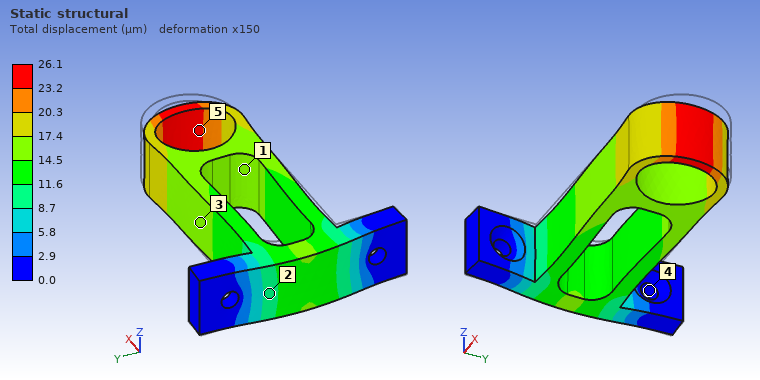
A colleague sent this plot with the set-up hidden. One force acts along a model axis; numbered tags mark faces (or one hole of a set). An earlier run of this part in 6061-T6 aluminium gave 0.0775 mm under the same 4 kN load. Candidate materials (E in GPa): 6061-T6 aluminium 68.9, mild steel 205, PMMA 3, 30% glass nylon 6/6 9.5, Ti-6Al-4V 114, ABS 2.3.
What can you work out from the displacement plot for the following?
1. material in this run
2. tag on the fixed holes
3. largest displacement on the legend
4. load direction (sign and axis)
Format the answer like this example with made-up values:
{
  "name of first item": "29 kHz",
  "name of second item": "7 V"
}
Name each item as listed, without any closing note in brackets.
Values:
{
  "material in this run": "mild steel",
  "tag on the fixed holes": "4",
  "largest displacement on the legend": "26.1 µm",
  "load direction": "-X"
}
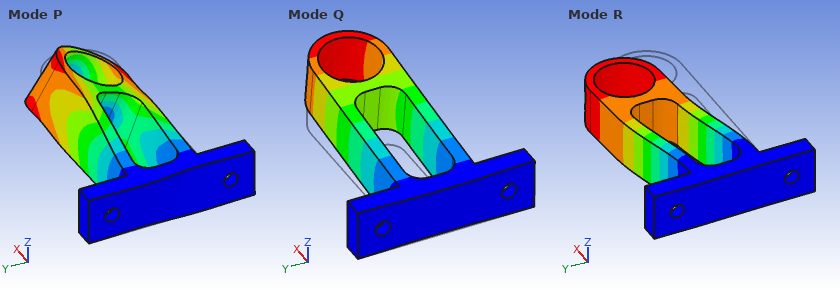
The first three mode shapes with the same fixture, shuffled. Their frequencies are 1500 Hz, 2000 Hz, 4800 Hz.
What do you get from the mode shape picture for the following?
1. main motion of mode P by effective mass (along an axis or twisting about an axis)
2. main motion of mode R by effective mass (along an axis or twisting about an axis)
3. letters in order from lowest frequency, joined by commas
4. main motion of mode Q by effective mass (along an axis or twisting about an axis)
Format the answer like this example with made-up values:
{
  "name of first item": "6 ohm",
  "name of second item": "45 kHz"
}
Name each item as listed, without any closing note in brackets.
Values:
{
  "main motion of mode P by effective mass": "twisting about X",
  "main motion of mode R by effective mass": "along Y",
  "letters in order from lowest frequency, joined by commas": "Q, R, P",
  "main motion of mode Q by effective mass": "along Z"
}
